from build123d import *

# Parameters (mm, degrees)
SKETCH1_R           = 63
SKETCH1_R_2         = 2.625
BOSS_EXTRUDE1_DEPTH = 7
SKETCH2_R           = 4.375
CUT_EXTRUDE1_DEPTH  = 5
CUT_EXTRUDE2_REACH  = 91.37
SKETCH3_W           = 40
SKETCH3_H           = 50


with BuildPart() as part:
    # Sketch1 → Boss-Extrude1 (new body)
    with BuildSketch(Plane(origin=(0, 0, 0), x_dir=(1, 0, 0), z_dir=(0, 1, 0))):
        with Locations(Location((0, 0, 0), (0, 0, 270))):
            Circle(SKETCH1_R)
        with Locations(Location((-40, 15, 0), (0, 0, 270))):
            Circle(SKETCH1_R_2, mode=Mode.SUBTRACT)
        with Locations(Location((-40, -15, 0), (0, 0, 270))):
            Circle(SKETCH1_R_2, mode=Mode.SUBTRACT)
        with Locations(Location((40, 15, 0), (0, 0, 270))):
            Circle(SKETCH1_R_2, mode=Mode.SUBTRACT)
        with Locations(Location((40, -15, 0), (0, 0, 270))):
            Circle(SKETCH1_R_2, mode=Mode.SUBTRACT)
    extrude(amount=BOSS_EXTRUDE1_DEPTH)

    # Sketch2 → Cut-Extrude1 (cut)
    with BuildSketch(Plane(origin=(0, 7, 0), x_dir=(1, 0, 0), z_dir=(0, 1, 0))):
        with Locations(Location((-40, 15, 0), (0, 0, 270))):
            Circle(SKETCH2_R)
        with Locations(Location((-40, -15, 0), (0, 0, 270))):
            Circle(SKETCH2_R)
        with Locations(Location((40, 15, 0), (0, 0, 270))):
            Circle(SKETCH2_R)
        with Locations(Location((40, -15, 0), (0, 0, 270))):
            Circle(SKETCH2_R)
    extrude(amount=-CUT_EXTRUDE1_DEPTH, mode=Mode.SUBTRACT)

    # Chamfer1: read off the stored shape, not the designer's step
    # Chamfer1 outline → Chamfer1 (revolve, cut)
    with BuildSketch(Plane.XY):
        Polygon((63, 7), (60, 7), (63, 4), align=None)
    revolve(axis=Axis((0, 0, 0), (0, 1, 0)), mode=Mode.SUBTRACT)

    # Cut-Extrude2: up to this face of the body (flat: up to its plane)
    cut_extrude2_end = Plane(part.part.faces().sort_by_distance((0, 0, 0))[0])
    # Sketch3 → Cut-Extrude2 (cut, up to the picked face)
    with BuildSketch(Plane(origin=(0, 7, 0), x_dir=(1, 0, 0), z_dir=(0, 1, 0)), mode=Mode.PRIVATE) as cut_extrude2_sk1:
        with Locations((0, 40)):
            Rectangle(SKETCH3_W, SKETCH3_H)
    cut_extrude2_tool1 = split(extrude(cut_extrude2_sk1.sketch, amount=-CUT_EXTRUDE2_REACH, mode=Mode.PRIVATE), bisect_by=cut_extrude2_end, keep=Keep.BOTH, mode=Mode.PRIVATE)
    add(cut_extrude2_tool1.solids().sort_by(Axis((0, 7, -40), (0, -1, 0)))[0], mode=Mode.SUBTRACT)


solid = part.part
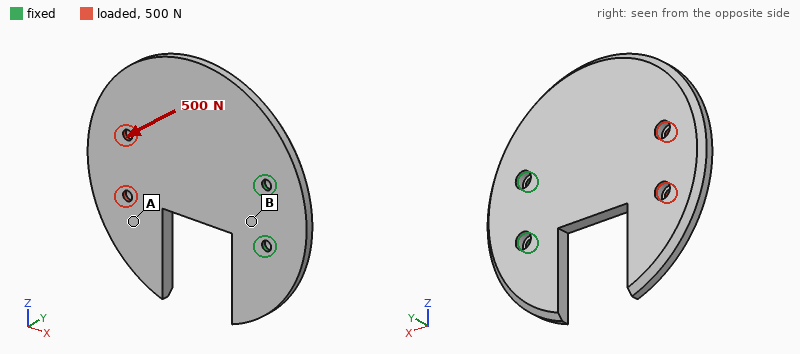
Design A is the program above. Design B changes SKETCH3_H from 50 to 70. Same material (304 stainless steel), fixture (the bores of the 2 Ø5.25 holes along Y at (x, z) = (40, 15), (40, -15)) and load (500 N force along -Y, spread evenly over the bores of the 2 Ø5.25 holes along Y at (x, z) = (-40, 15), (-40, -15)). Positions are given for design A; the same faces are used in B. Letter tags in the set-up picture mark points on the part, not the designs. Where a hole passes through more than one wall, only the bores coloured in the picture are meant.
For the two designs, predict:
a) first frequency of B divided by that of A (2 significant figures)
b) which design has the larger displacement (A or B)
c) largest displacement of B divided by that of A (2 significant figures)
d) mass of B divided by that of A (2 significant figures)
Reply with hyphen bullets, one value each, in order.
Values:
- 0.96
- B
- 1.1
- 0.96
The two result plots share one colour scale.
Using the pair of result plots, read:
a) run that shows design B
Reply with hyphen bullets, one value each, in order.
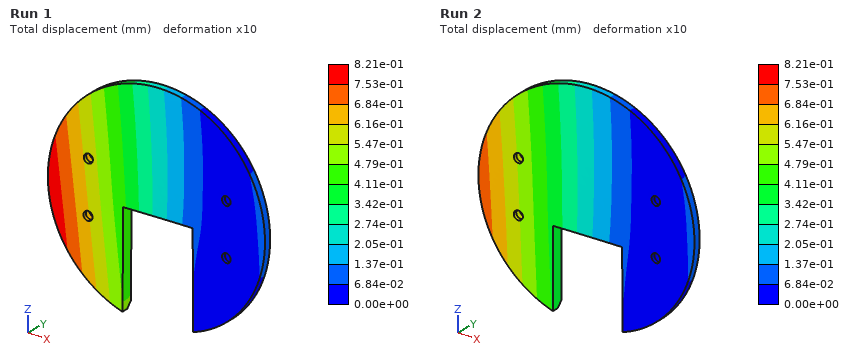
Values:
- Run 1
